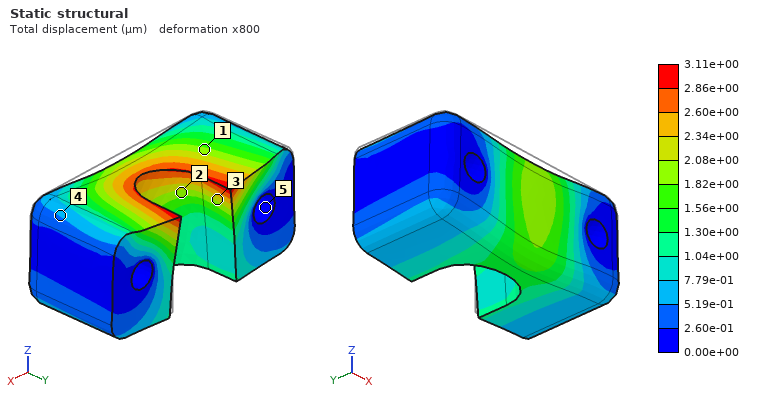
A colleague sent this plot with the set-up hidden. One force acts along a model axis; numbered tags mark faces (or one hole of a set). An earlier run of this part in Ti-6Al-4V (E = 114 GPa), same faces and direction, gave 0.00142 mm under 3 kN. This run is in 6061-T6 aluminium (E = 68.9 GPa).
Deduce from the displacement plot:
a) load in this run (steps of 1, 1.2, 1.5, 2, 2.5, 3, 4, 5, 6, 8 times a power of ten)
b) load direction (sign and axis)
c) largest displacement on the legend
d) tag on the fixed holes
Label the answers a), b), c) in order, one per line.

a) 4 kN
b) -Z
c) 3.11e+00 µm
d) 5
